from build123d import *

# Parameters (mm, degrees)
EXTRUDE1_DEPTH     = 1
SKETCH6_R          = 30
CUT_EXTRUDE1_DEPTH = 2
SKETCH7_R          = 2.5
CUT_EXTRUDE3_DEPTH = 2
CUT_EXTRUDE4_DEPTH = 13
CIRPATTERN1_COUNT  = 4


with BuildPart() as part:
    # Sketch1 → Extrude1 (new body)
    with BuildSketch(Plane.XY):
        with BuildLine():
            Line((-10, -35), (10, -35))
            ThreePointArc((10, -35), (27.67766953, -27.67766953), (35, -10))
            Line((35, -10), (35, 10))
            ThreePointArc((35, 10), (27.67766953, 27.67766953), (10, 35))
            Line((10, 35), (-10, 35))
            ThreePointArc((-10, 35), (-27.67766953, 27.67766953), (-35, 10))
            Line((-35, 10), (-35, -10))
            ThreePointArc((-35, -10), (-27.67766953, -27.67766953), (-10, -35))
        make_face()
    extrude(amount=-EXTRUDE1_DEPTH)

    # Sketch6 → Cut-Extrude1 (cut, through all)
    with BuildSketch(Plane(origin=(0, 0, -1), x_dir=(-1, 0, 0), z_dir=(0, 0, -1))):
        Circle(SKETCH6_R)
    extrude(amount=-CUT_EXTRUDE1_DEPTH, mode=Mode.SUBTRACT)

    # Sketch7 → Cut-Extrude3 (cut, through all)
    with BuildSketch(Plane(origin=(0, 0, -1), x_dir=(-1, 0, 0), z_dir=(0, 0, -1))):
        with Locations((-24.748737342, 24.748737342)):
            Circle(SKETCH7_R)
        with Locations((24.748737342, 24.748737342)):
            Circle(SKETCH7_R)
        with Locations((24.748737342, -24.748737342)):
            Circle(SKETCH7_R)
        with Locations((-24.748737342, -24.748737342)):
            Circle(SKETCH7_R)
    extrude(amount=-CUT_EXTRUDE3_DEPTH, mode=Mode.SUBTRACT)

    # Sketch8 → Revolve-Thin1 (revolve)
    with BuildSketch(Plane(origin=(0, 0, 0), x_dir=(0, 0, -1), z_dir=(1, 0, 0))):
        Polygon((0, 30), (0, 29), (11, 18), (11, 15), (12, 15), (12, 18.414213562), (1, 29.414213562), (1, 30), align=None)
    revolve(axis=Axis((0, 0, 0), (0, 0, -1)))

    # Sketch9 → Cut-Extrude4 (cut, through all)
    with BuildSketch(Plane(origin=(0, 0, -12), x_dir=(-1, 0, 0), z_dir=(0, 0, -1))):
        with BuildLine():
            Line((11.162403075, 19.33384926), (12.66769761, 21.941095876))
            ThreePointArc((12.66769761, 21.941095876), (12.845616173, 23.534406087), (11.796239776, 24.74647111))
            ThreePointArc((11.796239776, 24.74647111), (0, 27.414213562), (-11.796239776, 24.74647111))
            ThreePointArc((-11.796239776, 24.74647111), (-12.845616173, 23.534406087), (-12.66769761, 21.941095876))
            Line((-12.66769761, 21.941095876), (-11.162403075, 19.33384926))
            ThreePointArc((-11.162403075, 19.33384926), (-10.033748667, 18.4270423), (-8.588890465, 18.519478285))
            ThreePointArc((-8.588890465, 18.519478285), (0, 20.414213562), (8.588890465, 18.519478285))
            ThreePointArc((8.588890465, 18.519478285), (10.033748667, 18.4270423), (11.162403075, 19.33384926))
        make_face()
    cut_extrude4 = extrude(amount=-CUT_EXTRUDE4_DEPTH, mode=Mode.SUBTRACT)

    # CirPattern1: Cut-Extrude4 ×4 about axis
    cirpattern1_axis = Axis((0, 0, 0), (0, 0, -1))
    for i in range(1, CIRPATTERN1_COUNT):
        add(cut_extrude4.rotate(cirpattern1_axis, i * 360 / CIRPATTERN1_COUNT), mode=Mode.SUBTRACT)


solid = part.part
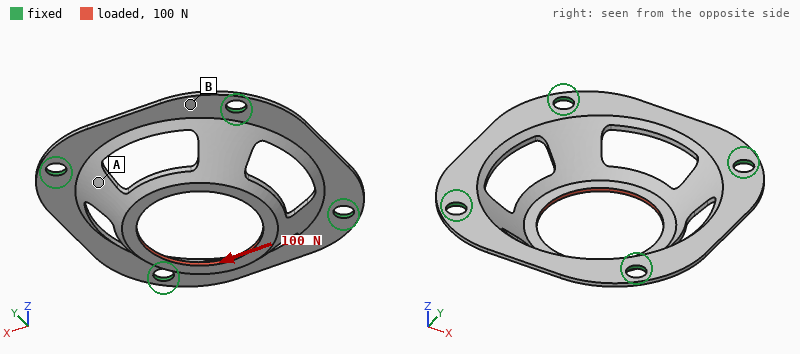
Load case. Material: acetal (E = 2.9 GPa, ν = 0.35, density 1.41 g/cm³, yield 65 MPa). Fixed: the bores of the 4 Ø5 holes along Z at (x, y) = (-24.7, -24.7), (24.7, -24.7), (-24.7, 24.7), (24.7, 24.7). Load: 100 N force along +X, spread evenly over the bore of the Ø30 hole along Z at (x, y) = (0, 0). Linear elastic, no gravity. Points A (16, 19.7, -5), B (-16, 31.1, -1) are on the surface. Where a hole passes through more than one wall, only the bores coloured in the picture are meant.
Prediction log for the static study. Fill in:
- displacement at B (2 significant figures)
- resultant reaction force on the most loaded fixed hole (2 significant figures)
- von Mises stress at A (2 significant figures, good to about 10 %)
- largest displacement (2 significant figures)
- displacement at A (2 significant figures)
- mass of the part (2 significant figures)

0.093 mm
27 N
8.8 MPa
0.43 mm
0.13 mm
4.6 g
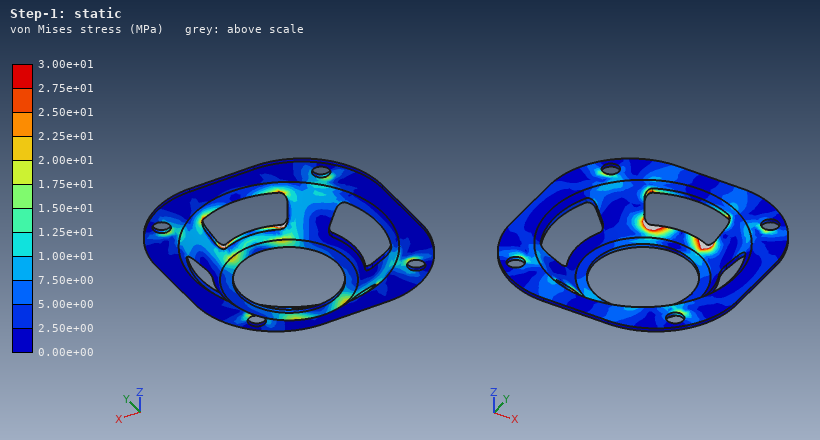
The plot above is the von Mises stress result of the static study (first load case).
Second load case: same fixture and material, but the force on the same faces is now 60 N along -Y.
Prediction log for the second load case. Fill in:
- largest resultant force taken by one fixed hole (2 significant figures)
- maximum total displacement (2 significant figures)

16 N
0.26 mm
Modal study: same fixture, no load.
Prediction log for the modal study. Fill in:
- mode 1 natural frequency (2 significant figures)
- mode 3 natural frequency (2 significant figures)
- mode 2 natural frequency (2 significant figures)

1300 Hz
1300 Hz
1300 Hz
